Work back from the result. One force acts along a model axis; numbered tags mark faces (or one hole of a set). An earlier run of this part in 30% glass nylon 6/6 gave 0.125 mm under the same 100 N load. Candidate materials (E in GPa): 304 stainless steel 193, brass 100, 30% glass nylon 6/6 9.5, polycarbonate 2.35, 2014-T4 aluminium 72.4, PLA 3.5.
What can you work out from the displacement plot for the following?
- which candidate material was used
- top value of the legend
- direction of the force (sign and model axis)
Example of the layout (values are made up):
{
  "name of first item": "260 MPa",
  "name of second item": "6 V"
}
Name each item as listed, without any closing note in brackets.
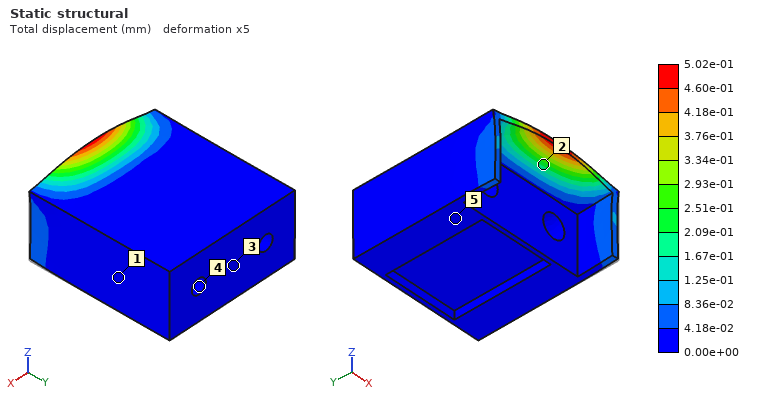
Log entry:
{
  "which candidate material was used": "polycarbonate",
  "top value of the legend": "5.02e-01 mm",
  "direction of the force": "+Z"
}
